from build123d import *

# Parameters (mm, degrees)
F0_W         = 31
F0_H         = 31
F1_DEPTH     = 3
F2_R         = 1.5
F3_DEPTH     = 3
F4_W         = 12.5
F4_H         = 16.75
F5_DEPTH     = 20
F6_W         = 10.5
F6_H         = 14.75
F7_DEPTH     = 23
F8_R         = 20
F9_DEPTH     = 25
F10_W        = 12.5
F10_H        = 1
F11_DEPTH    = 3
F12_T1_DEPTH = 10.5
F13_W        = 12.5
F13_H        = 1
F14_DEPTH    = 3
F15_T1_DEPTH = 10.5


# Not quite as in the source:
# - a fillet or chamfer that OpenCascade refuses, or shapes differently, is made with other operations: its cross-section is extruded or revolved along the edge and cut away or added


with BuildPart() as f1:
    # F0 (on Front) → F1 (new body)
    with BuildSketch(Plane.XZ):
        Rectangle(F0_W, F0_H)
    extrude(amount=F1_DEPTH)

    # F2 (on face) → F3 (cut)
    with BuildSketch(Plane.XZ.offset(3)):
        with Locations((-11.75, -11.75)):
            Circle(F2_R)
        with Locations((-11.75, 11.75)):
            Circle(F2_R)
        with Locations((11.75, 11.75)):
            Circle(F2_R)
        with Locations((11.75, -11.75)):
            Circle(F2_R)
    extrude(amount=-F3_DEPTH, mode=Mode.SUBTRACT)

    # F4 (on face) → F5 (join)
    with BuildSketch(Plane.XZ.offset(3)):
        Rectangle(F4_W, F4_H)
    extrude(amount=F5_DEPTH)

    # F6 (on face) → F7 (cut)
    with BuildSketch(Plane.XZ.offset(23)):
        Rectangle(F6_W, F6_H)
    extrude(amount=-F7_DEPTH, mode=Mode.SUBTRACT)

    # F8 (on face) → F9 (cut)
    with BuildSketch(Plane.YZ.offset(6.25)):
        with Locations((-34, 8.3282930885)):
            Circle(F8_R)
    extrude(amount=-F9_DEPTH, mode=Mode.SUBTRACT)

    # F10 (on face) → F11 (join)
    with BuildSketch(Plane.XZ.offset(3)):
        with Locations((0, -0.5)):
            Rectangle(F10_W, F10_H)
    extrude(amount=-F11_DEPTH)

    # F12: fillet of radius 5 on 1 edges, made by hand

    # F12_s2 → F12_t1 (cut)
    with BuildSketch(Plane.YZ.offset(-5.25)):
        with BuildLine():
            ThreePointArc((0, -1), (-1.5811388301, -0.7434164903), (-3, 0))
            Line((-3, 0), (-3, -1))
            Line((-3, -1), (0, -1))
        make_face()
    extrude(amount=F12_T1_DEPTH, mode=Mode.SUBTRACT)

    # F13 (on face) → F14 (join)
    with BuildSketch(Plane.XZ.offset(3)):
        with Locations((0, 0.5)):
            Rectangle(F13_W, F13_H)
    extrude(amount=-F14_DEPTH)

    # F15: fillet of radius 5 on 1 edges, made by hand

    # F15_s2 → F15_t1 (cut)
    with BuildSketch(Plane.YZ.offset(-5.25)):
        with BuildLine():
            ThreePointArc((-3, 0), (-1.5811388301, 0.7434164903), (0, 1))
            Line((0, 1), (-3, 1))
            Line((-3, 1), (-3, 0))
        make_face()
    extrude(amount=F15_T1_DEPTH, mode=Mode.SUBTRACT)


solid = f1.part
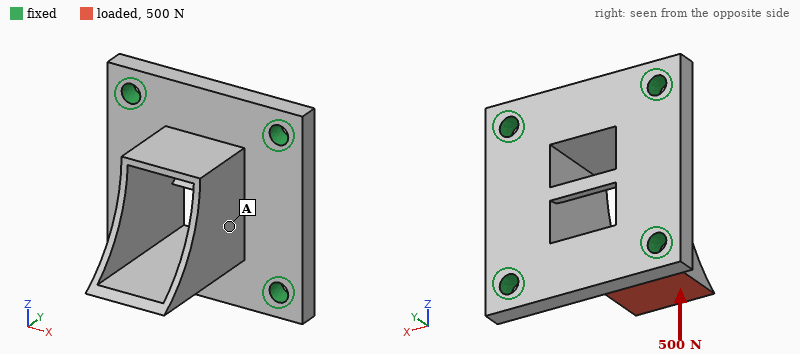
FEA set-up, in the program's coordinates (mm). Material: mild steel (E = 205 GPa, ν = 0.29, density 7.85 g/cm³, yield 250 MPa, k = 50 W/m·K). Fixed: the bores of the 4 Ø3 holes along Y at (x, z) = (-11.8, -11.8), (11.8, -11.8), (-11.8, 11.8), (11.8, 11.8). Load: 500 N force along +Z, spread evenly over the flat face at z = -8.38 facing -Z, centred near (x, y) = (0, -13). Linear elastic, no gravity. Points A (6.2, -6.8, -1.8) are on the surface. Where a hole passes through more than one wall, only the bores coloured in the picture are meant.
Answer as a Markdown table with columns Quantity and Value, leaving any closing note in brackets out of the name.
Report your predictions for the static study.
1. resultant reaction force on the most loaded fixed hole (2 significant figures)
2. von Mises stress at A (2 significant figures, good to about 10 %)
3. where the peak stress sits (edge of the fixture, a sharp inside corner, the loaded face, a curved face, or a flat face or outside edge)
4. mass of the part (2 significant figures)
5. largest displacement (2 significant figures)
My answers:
| Quantity | Value |
|---|---|
| resultant reaction force on the most loaded fixed hole | 200 N |
| von Mises stress at A | 22 MPa |
| where the peak stress sits | a curved face |
| mass of the part | 25 g |
| largest displacement | 38 µm |
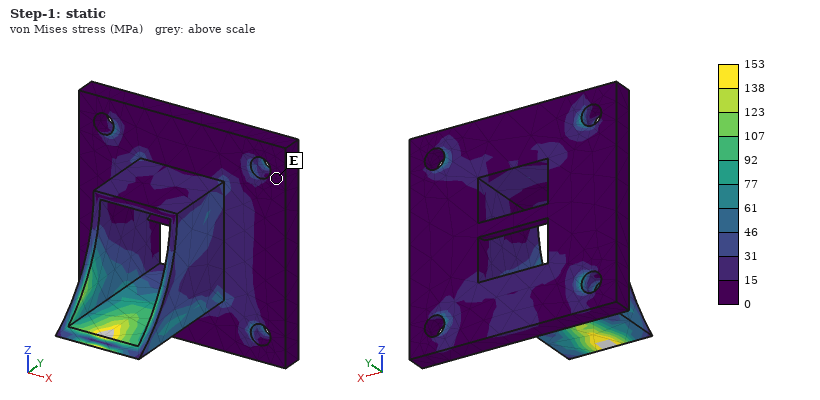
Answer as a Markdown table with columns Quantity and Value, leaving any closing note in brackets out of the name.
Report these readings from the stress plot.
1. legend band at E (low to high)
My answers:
| Quantity | Value |
|---|---|
| legend band at E | 0 to 15 MPa |
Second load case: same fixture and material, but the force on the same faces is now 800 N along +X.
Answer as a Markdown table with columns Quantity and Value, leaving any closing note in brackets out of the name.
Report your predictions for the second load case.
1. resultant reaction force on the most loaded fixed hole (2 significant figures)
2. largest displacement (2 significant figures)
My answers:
| Quantity | Value |
|---|---|
| resultant reaction force on the most loaded fixed hole | 560 N |
| largest displacement | 41 µm |
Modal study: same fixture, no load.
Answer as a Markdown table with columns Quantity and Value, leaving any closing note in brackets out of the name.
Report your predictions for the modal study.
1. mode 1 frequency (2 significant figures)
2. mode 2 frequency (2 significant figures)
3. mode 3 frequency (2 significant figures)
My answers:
| Quantity | Value |
|---|---|
| mode 1 frequency | 14 kHz |
| mode 2 frequency | 15 kHz |
| mode 3 frequency | 18 kHz |
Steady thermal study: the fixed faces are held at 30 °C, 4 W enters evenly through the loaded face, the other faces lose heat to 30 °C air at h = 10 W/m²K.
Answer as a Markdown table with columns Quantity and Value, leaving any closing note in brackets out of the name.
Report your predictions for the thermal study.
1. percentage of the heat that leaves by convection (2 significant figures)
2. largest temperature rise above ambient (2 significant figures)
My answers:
| Quantity | Value |
|---|---|
| percentage of the heat that leaves by convection | 5.9 % |
| largest temperature rise above ambient | 36 K |
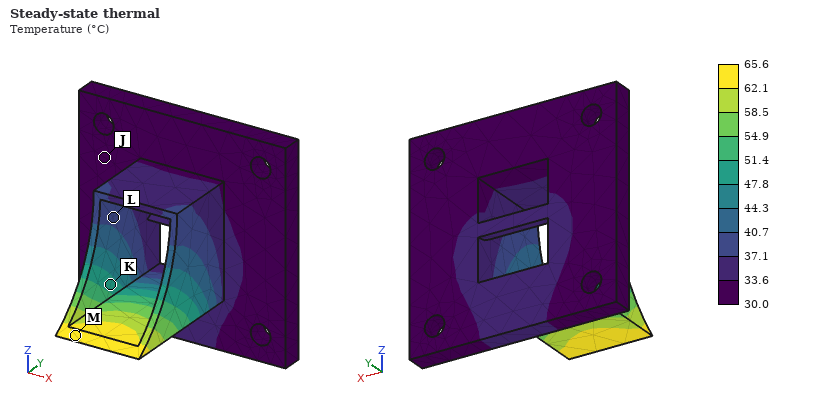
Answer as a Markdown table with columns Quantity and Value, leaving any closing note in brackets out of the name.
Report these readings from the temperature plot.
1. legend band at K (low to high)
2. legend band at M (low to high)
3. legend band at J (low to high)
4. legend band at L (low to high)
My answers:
| Quantity | Value |
|---|---|
| legend band at K | 47.8 to 51.4 °C |
| legend band at M | 62.1 to 65.6 °C |
| legend band at J | 30.0 to 33.6 °C |
| legend band at L | 37.1 to 40.7 °C |
